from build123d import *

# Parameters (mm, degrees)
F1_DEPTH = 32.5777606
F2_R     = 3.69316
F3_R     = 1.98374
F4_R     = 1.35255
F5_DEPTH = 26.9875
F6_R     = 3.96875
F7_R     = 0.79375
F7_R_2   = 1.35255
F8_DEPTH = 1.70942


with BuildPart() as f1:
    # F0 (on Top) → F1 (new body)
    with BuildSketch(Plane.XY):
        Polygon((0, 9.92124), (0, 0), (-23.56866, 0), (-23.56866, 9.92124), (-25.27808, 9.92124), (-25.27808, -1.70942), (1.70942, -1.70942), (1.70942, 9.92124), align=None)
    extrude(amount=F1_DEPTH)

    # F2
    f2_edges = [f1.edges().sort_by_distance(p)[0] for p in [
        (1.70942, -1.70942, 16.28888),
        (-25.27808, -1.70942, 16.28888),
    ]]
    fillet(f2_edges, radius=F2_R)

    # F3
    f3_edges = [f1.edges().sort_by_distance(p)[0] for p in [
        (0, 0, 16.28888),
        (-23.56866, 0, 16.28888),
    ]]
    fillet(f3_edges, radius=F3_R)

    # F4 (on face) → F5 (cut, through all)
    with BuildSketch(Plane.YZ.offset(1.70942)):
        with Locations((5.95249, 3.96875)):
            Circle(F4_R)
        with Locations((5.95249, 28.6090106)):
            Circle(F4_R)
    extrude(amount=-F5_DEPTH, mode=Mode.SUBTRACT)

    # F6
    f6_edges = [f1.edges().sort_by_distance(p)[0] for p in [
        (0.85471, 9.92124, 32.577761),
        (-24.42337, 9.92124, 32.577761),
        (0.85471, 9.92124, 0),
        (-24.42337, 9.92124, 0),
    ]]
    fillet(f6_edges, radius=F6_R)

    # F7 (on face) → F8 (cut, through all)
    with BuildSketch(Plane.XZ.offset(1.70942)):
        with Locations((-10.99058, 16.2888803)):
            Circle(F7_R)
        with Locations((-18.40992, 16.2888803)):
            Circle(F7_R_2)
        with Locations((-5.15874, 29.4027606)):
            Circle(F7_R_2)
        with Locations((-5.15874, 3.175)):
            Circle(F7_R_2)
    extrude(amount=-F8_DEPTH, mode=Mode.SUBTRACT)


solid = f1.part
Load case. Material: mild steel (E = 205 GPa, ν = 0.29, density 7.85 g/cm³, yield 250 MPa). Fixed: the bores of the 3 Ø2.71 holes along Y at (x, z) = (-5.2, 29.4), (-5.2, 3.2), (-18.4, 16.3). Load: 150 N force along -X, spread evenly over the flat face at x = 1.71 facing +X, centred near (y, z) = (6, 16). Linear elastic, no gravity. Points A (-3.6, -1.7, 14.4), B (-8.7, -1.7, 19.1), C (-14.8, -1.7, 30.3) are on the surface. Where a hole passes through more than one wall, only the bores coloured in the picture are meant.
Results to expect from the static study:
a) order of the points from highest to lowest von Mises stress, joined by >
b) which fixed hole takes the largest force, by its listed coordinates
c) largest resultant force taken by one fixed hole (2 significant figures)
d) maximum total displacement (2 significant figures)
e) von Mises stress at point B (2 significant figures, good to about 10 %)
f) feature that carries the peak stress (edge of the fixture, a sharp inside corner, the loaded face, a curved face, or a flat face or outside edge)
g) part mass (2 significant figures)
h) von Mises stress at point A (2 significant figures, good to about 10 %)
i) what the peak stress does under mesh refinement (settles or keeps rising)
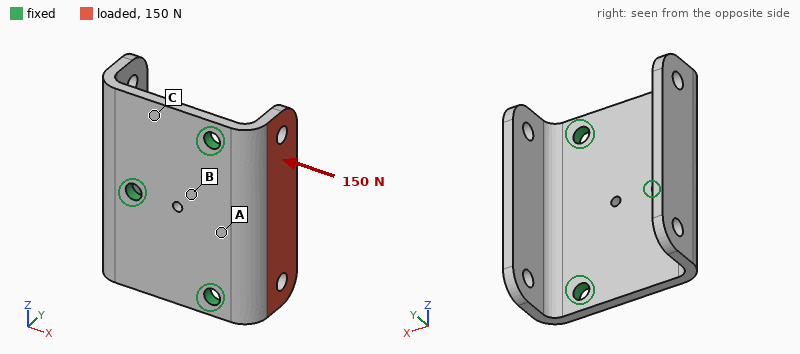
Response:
A > B > C
(-18.4, 16.3)
59 N
31 µm
13 MPa
edge of the fixture
19 g
38 MPa
keeps rising
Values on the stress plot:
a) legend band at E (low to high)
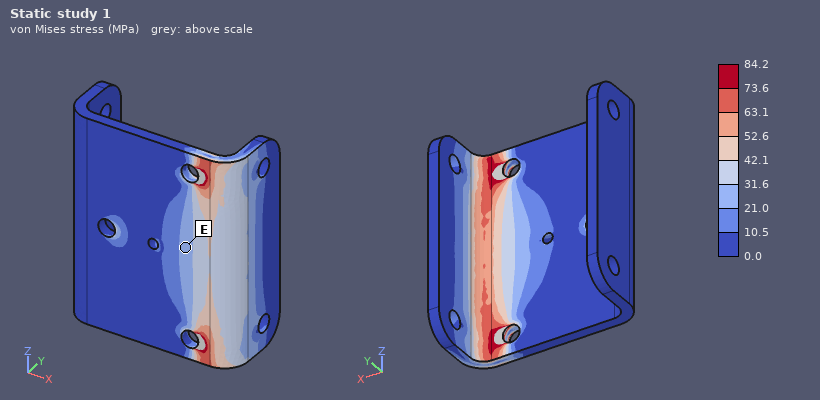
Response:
21.0 to 31.6 MPa
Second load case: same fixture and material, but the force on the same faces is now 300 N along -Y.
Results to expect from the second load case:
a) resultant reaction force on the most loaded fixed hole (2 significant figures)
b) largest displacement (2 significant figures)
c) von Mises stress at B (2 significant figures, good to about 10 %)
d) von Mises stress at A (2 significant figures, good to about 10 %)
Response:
170 N
34 µm
20 MPa
38 MPa
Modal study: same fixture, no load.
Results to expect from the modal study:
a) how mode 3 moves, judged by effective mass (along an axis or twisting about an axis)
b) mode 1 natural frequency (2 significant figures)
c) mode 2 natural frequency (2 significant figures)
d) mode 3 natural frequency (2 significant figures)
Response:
along X
5300 Hz
6400 Hz
7000 Hz
